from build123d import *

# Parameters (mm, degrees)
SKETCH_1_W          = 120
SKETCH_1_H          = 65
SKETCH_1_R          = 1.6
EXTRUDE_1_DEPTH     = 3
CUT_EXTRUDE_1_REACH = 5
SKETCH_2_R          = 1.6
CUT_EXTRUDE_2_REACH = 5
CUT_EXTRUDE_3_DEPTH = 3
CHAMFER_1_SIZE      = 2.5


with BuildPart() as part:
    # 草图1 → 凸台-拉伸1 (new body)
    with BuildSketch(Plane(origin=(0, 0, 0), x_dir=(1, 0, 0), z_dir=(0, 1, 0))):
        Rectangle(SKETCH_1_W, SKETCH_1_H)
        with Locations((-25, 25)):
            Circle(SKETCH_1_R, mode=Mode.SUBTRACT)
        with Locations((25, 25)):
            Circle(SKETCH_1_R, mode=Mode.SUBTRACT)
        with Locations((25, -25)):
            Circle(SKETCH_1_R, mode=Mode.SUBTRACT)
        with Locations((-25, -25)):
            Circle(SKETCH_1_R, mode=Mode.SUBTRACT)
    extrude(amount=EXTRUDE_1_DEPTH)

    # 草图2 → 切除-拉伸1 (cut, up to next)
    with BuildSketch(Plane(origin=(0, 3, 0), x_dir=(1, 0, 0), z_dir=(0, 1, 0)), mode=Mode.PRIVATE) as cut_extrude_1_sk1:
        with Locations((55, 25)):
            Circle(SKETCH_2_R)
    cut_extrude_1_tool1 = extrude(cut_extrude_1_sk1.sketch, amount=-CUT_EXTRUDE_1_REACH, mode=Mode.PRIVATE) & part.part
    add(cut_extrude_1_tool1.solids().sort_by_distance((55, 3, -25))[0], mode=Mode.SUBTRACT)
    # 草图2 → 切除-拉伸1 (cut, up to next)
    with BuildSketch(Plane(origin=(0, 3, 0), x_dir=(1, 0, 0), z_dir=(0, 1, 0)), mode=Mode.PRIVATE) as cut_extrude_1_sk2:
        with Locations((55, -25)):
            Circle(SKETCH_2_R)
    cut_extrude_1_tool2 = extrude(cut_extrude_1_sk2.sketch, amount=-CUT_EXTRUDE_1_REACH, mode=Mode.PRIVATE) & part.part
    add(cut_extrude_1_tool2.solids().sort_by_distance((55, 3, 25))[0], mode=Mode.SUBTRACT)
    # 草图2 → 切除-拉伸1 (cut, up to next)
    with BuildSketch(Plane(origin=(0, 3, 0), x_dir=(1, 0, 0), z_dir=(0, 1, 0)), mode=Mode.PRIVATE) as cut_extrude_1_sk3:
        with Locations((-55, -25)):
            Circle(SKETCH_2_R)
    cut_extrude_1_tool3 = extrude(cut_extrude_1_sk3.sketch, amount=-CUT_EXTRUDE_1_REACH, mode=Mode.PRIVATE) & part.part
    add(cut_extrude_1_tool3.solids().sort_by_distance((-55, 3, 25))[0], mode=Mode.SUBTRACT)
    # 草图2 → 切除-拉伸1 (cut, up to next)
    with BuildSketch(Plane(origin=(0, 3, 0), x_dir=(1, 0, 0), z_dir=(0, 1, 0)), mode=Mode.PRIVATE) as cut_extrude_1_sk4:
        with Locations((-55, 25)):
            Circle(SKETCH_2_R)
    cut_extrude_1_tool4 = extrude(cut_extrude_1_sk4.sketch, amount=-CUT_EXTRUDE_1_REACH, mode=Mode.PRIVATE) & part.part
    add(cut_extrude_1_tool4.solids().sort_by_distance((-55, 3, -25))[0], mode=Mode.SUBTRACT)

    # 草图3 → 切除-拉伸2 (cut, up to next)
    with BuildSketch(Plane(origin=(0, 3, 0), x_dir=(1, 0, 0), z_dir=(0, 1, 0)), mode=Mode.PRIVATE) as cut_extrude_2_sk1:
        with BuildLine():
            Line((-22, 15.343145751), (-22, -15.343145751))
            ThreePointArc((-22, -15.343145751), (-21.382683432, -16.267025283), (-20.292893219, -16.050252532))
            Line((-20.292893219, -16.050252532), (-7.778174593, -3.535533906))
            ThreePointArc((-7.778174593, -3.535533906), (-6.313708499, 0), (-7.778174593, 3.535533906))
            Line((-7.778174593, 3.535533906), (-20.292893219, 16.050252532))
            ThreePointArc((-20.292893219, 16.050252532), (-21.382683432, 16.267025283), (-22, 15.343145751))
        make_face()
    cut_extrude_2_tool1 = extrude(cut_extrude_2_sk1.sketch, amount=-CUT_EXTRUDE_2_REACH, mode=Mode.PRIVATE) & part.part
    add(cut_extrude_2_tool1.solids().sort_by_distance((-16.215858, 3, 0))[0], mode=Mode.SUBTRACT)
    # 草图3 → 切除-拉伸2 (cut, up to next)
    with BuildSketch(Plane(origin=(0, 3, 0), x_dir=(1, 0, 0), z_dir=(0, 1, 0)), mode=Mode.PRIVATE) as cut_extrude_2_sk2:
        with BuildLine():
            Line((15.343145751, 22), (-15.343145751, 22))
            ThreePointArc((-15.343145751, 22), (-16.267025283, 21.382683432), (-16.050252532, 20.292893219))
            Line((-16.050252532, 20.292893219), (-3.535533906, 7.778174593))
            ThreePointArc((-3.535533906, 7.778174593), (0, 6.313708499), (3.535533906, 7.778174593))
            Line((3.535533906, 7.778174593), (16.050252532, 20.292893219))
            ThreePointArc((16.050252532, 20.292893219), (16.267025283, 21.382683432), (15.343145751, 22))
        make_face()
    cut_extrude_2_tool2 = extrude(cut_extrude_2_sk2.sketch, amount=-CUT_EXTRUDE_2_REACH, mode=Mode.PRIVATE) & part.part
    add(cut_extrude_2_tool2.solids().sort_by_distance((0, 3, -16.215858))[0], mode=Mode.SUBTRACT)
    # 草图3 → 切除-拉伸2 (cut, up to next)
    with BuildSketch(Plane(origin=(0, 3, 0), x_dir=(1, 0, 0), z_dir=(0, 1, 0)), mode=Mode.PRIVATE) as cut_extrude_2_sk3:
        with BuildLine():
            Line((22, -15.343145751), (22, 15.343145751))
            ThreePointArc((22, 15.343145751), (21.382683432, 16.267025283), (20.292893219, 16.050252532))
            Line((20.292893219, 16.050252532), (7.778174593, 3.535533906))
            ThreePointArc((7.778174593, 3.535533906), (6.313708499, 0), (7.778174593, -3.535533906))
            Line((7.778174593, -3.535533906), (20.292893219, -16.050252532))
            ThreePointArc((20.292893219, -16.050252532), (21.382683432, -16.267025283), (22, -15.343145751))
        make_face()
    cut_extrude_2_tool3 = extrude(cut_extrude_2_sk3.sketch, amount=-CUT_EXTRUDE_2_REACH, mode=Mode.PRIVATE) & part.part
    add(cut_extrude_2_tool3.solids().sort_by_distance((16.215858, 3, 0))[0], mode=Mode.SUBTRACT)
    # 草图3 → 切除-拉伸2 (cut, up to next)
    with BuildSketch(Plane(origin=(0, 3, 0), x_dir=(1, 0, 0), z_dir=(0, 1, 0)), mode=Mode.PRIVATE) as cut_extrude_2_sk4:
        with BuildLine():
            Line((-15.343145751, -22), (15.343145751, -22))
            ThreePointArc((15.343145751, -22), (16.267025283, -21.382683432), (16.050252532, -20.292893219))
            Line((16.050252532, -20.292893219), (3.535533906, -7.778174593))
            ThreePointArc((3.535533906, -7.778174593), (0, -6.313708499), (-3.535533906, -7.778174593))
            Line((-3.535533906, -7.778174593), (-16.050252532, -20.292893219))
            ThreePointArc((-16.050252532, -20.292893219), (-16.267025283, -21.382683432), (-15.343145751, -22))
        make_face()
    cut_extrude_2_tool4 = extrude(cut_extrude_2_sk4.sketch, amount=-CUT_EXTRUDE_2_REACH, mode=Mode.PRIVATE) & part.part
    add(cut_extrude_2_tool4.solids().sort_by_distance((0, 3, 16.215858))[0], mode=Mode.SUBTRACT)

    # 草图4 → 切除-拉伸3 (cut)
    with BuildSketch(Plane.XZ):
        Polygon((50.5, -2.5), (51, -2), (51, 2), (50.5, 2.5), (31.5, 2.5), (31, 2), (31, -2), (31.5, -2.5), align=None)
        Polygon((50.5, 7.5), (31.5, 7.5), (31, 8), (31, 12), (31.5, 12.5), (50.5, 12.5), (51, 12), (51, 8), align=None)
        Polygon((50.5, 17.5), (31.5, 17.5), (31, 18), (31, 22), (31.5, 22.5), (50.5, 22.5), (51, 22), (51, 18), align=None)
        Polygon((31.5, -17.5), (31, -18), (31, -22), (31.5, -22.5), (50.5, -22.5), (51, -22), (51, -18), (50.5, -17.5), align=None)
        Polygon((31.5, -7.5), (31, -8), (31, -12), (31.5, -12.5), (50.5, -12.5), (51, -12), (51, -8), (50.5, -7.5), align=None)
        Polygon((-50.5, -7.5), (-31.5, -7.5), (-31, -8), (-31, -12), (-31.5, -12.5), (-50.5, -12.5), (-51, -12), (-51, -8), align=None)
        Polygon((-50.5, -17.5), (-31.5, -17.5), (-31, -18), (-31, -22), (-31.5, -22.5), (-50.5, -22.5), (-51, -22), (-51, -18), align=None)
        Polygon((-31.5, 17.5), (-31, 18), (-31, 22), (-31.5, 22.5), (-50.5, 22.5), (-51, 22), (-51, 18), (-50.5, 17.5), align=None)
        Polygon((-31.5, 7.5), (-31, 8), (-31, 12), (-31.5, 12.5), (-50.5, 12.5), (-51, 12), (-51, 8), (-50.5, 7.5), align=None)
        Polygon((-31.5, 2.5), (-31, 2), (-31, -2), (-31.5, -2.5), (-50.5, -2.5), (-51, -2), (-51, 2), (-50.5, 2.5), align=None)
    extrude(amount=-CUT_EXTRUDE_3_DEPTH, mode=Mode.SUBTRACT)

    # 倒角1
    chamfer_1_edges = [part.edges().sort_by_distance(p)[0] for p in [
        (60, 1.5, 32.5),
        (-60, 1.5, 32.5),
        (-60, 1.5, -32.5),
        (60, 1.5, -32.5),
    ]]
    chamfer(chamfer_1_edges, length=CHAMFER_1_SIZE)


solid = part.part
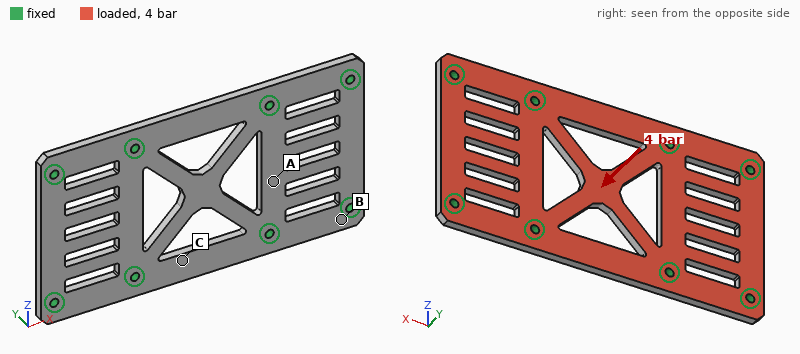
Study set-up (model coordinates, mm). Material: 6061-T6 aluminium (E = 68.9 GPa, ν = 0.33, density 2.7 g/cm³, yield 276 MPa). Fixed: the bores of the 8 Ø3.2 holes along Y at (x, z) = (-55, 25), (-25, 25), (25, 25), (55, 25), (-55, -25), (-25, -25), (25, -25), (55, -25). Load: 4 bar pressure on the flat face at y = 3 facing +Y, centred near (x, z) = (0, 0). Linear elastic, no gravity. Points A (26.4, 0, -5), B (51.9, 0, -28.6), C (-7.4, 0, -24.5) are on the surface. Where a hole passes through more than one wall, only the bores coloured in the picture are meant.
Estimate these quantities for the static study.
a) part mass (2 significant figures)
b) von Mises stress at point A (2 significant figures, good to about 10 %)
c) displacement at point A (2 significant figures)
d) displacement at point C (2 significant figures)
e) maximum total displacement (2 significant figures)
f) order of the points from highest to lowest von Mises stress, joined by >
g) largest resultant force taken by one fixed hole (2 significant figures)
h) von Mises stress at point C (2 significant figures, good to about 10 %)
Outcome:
45 g
31 MPa
0.052 mm
0.033 mm
0.10 mm
A > C > B
360 N
17 MPa
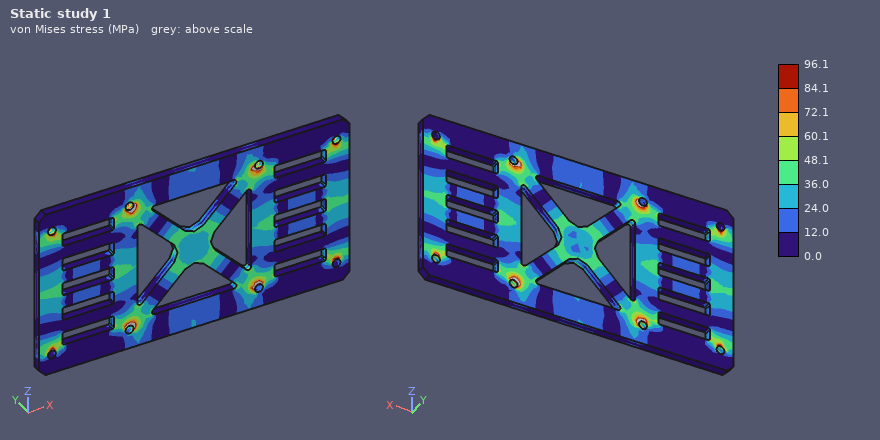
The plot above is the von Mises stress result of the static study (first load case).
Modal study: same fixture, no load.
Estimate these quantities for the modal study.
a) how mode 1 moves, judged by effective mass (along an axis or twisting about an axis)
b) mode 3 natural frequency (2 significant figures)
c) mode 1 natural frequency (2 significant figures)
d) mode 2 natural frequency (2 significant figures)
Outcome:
along Y
5300 Hz
4200 Hz
5300 Hz
